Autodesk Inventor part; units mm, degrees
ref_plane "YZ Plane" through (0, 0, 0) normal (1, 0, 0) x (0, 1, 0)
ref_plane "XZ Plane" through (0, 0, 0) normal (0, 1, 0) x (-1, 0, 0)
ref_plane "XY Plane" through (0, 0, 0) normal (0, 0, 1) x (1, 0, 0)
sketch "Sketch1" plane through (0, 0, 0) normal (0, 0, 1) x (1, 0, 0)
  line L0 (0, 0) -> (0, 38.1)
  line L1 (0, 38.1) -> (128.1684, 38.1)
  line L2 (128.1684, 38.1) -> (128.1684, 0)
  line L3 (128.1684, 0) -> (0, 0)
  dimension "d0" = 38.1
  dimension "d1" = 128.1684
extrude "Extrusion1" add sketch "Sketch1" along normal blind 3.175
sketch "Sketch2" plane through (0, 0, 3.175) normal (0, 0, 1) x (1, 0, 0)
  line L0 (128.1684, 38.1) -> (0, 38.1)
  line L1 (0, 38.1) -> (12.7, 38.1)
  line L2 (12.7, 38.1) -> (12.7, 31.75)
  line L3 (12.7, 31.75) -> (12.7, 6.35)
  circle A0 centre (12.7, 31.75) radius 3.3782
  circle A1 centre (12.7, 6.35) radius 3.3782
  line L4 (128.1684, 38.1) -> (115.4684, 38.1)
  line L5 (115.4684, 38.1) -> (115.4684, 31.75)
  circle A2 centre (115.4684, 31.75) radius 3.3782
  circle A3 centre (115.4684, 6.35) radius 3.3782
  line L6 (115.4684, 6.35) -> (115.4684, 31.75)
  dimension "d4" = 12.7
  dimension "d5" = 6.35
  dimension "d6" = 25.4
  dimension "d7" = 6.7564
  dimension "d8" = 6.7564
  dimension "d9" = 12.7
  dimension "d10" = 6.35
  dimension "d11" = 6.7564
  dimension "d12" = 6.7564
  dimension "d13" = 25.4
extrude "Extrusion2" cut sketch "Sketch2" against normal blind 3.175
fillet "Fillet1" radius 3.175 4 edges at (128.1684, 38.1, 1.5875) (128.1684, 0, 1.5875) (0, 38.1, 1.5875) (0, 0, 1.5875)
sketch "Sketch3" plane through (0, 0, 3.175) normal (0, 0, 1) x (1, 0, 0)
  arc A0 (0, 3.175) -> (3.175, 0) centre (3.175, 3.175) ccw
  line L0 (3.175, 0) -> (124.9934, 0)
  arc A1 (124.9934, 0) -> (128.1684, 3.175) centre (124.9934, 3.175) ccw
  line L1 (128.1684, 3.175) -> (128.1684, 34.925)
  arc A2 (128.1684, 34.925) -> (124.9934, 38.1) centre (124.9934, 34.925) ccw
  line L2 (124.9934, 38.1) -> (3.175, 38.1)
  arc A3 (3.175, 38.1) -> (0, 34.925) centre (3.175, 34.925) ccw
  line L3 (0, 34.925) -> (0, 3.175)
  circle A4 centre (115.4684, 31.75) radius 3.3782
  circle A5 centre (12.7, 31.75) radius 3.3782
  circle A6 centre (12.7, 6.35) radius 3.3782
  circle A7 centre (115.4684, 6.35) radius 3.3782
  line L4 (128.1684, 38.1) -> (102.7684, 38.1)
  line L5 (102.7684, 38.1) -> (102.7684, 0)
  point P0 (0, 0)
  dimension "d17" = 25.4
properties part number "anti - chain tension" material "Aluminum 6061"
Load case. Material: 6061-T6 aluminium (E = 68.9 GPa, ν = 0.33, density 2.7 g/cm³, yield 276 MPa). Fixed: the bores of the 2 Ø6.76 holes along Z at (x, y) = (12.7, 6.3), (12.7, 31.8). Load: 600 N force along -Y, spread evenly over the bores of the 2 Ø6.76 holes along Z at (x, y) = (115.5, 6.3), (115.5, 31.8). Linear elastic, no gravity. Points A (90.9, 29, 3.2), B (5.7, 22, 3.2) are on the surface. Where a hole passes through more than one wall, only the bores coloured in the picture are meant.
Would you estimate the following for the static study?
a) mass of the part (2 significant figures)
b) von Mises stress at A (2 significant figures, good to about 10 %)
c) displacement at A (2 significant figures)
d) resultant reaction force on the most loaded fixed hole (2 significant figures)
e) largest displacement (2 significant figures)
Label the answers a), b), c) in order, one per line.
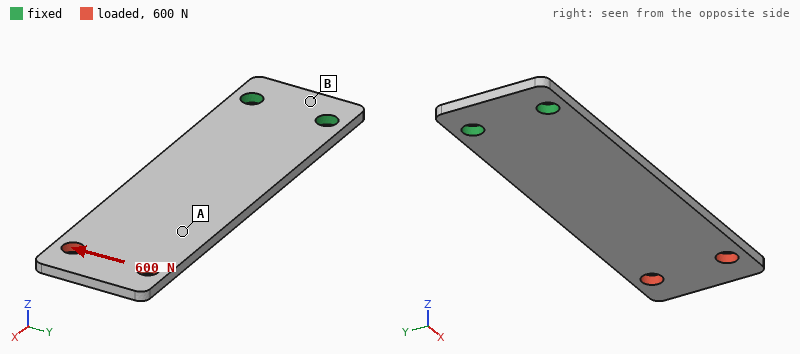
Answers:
a) 41 g
b) 14 MPa
c) 0.15 mm
d) 2.2 kN
e) 0.27 mm
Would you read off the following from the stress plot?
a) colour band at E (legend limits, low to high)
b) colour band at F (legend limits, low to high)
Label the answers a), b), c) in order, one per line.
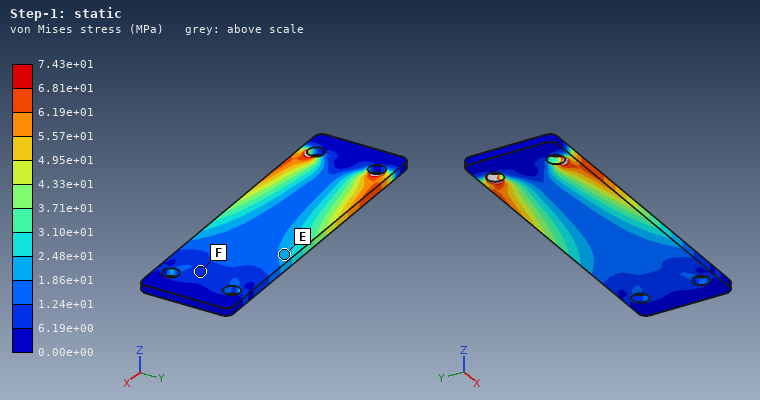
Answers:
a) 1.86e+01 to 2.48e+01 MPa
b) 6.19e+00 to 1.24e+01 MPa
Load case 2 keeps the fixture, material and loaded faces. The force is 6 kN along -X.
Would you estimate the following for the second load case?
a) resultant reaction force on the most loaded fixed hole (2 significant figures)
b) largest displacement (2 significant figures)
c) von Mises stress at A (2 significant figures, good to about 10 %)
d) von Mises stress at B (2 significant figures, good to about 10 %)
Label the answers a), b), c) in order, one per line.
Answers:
a) 3.0 kN
b) 83 µm
c) 49 MPa
d) 13 MPa
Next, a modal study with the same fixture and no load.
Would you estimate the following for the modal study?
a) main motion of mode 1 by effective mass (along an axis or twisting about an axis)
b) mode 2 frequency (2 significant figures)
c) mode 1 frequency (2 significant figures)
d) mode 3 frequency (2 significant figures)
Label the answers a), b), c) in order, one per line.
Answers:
a) along Z
b) 1200 Hz
c) 210 Hz
d) 1300 Hz
